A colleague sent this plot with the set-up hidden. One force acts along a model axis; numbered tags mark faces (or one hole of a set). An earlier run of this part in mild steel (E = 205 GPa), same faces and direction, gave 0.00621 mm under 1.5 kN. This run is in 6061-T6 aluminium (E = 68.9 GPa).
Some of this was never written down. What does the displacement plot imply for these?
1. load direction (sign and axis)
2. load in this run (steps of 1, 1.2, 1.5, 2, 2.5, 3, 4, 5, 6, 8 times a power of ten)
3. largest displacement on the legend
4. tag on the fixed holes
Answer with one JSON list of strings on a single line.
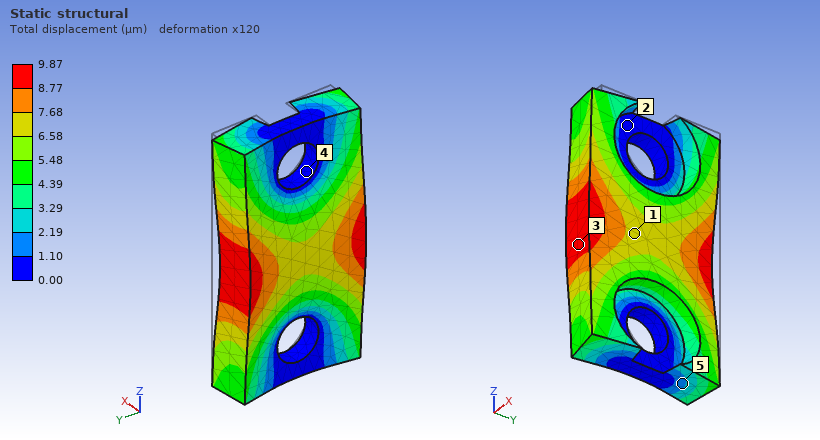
["-X", "800 N", "9.87 µm", "4"]
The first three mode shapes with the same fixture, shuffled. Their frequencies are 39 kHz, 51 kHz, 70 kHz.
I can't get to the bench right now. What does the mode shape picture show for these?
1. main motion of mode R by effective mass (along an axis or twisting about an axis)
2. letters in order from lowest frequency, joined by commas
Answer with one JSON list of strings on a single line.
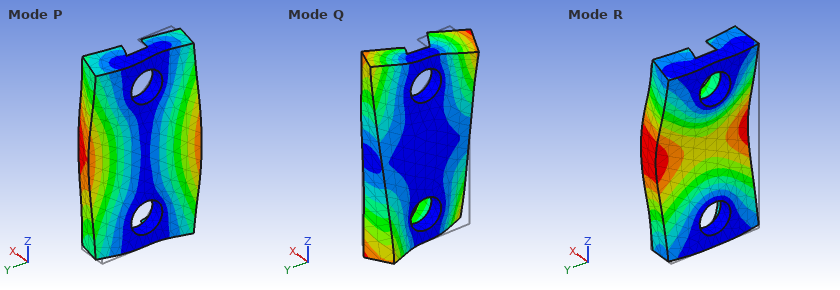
["along X", "P, R, Q"]
